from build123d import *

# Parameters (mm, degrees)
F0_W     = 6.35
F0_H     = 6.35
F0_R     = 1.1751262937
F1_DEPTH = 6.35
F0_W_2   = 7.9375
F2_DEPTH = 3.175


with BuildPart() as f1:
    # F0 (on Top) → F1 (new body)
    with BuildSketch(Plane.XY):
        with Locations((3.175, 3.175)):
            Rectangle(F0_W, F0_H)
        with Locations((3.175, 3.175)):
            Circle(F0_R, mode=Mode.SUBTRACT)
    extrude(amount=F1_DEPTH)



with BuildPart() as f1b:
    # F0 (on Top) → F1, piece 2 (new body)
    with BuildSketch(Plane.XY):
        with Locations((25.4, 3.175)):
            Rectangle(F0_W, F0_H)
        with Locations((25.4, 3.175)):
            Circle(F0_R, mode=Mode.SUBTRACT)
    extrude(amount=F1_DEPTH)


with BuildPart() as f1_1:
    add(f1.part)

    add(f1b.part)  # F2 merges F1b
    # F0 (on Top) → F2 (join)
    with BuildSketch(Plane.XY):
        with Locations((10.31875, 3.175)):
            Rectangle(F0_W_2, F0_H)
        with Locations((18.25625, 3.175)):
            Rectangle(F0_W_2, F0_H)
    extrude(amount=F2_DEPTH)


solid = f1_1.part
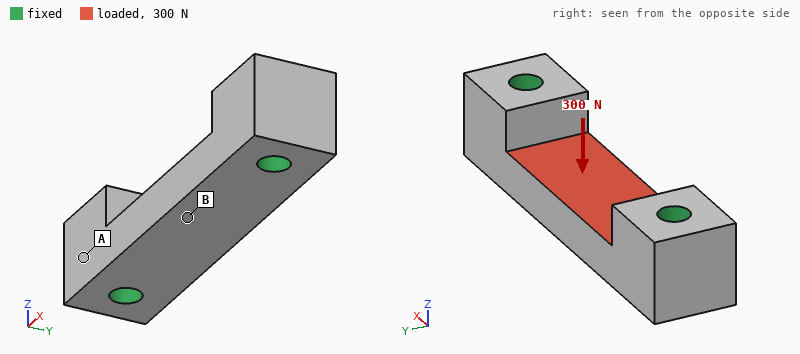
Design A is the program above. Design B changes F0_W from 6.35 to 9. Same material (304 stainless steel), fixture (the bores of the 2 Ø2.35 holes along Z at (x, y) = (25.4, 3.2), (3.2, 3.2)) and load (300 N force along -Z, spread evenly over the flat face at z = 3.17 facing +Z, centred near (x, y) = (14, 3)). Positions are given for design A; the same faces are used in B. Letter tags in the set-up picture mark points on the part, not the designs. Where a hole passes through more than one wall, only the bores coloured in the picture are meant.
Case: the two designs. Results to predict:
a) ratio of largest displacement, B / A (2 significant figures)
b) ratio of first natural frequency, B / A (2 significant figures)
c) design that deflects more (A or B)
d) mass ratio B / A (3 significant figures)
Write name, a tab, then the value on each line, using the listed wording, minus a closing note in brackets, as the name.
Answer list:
ratio of largest displacement, B / A	0.83
ratio of first natural frequency, B / A	1.2
design that deflects more	A
mass ratio B / A	1.21
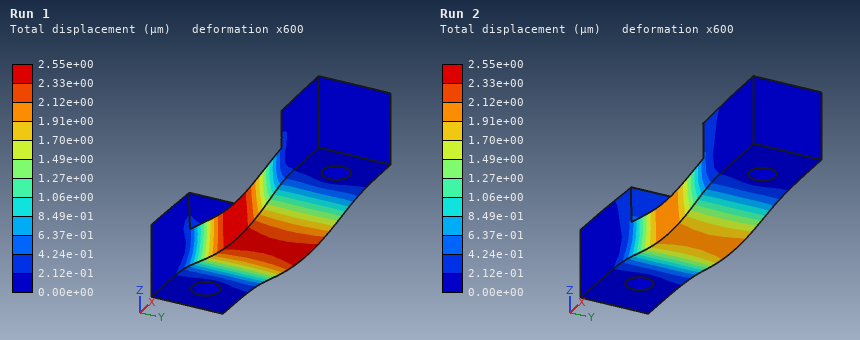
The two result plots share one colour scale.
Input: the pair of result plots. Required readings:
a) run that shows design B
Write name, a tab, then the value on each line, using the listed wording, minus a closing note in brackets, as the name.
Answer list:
run that shows design B	Run 2
